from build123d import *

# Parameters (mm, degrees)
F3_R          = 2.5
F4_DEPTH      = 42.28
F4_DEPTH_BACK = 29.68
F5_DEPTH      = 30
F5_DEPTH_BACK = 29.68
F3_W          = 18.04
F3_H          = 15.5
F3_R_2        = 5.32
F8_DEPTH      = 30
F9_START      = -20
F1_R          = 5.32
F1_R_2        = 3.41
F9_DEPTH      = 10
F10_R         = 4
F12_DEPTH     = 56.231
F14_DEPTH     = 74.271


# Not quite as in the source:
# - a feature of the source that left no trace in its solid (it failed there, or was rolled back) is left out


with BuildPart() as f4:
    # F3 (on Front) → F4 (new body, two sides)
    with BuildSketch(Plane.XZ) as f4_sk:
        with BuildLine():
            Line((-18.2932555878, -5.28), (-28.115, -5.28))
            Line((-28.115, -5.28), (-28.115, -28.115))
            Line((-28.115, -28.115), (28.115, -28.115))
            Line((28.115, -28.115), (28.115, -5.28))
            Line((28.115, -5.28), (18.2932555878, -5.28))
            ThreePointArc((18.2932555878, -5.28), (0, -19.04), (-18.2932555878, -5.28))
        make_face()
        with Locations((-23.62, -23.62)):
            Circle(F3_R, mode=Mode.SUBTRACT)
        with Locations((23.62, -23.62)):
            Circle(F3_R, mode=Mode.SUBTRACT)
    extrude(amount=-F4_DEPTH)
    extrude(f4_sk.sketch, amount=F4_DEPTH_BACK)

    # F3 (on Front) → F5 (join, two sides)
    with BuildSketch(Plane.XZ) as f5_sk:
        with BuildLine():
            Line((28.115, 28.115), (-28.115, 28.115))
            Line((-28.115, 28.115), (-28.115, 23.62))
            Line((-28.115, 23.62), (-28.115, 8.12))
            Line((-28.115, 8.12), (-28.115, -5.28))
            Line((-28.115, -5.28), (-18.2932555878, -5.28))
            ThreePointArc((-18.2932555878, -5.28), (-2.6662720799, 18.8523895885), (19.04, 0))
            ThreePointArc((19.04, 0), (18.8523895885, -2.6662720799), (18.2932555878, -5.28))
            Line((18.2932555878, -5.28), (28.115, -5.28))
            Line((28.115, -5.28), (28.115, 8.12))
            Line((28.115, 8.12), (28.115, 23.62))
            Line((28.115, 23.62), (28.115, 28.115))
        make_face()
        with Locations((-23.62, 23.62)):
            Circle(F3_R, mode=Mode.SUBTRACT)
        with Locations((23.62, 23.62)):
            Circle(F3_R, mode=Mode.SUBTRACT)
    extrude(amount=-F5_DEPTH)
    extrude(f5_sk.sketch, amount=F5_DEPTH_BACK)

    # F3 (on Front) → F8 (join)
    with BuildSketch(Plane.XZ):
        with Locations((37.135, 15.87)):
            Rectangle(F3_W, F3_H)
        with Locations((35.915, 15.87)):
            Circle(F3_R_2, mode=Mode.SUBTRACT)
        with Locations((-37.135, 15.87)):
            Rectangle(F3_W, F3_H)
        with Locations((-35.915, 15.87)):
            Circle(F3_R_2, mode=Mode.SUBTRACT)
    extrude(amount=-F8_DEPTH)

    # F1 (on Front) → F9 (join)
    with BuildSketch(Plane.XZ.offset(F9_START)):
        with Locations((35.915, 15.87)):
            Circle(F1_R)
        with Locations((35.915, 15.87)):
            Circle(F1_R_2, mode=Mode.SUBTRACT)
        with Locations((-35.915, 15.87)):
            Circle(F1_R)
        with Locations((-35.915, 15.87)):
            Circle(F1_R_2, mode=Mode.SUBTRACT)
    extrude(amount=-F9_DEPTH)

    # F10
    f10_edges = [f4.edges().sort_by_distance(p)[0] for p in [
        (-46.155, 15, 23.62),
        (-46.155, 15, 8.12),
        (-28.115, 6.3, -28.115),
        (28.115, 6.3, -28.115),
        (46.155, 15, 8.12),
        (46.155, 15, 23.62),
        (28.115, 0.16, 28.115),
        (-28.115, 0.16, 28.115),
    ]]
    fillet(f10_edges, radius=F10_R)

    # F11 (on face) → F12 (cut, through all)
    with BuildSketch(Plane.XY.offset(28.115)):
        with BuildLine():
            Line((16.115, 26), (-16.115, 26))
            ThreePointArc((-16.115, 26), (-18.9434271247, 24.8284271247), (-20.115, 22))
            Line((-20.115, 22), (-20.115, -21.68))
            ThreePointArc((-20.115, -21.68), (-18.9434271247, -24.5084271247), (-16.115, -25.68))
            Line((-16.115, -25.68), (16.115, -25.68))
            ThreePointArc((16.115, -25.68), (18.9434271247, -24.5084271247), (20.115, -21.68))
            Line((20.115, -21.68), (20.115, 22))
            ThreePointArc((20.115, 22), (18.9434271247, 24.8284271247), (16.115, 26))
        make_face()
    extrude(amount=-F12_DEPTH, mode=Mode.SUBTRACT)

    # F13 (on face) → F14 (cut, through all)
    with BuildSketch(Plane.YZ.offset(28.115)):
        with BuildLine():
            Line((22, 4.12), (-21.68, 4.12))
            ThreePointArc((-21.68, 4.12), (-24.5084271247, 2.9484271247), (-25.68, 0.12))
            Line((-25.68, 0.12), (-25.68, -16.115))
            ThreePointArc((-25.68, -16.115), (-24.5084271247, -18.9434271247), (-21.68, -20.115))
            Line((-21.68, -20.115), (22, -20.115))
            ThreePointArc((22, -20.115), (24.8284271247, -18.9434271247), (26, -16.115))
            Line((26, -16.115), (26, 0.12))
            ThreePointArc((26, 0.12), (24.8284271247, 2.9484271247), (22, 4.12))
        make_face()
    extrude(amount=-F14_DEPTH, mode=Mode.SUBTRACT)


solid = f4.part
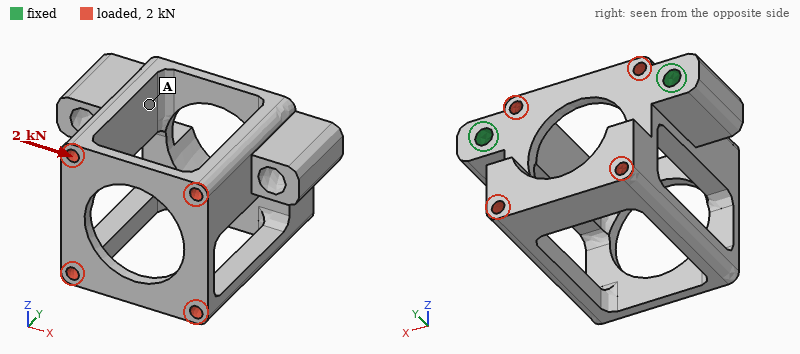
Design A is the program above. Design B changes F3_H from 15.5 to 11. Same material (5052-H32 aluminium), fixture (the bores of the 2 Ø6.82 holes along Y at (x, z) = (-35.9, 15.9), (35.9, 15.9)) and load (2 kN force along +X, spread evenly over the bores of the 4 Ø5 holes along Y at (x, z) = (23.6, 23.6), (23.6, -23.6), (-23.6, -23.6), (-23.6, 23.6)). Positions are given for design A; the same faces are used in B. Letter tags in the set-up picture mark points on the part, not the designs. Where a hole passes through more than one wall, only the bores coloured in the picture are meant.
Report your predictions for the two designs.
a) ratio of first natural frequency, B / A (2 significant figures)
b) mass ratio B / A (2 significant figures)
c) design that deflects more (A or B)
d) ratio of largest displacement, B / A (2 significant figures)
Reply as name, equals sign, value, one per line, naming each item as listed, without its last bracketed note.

ratio of first natural frequency, B / A = 0.82
mass ratio B / A = 0.92
design that deflects more = B
ratio of largest displacement, B / A = 1.2
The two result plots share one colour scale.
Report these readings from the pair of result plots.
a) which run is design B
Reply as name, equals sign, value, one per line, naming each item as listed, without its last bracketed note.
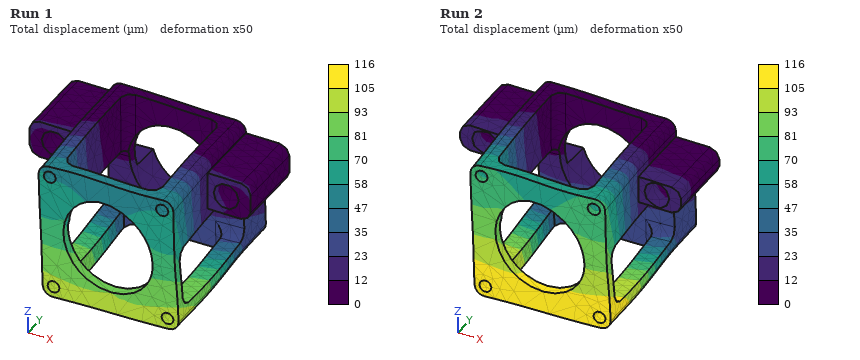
which run is design B = Run 2
